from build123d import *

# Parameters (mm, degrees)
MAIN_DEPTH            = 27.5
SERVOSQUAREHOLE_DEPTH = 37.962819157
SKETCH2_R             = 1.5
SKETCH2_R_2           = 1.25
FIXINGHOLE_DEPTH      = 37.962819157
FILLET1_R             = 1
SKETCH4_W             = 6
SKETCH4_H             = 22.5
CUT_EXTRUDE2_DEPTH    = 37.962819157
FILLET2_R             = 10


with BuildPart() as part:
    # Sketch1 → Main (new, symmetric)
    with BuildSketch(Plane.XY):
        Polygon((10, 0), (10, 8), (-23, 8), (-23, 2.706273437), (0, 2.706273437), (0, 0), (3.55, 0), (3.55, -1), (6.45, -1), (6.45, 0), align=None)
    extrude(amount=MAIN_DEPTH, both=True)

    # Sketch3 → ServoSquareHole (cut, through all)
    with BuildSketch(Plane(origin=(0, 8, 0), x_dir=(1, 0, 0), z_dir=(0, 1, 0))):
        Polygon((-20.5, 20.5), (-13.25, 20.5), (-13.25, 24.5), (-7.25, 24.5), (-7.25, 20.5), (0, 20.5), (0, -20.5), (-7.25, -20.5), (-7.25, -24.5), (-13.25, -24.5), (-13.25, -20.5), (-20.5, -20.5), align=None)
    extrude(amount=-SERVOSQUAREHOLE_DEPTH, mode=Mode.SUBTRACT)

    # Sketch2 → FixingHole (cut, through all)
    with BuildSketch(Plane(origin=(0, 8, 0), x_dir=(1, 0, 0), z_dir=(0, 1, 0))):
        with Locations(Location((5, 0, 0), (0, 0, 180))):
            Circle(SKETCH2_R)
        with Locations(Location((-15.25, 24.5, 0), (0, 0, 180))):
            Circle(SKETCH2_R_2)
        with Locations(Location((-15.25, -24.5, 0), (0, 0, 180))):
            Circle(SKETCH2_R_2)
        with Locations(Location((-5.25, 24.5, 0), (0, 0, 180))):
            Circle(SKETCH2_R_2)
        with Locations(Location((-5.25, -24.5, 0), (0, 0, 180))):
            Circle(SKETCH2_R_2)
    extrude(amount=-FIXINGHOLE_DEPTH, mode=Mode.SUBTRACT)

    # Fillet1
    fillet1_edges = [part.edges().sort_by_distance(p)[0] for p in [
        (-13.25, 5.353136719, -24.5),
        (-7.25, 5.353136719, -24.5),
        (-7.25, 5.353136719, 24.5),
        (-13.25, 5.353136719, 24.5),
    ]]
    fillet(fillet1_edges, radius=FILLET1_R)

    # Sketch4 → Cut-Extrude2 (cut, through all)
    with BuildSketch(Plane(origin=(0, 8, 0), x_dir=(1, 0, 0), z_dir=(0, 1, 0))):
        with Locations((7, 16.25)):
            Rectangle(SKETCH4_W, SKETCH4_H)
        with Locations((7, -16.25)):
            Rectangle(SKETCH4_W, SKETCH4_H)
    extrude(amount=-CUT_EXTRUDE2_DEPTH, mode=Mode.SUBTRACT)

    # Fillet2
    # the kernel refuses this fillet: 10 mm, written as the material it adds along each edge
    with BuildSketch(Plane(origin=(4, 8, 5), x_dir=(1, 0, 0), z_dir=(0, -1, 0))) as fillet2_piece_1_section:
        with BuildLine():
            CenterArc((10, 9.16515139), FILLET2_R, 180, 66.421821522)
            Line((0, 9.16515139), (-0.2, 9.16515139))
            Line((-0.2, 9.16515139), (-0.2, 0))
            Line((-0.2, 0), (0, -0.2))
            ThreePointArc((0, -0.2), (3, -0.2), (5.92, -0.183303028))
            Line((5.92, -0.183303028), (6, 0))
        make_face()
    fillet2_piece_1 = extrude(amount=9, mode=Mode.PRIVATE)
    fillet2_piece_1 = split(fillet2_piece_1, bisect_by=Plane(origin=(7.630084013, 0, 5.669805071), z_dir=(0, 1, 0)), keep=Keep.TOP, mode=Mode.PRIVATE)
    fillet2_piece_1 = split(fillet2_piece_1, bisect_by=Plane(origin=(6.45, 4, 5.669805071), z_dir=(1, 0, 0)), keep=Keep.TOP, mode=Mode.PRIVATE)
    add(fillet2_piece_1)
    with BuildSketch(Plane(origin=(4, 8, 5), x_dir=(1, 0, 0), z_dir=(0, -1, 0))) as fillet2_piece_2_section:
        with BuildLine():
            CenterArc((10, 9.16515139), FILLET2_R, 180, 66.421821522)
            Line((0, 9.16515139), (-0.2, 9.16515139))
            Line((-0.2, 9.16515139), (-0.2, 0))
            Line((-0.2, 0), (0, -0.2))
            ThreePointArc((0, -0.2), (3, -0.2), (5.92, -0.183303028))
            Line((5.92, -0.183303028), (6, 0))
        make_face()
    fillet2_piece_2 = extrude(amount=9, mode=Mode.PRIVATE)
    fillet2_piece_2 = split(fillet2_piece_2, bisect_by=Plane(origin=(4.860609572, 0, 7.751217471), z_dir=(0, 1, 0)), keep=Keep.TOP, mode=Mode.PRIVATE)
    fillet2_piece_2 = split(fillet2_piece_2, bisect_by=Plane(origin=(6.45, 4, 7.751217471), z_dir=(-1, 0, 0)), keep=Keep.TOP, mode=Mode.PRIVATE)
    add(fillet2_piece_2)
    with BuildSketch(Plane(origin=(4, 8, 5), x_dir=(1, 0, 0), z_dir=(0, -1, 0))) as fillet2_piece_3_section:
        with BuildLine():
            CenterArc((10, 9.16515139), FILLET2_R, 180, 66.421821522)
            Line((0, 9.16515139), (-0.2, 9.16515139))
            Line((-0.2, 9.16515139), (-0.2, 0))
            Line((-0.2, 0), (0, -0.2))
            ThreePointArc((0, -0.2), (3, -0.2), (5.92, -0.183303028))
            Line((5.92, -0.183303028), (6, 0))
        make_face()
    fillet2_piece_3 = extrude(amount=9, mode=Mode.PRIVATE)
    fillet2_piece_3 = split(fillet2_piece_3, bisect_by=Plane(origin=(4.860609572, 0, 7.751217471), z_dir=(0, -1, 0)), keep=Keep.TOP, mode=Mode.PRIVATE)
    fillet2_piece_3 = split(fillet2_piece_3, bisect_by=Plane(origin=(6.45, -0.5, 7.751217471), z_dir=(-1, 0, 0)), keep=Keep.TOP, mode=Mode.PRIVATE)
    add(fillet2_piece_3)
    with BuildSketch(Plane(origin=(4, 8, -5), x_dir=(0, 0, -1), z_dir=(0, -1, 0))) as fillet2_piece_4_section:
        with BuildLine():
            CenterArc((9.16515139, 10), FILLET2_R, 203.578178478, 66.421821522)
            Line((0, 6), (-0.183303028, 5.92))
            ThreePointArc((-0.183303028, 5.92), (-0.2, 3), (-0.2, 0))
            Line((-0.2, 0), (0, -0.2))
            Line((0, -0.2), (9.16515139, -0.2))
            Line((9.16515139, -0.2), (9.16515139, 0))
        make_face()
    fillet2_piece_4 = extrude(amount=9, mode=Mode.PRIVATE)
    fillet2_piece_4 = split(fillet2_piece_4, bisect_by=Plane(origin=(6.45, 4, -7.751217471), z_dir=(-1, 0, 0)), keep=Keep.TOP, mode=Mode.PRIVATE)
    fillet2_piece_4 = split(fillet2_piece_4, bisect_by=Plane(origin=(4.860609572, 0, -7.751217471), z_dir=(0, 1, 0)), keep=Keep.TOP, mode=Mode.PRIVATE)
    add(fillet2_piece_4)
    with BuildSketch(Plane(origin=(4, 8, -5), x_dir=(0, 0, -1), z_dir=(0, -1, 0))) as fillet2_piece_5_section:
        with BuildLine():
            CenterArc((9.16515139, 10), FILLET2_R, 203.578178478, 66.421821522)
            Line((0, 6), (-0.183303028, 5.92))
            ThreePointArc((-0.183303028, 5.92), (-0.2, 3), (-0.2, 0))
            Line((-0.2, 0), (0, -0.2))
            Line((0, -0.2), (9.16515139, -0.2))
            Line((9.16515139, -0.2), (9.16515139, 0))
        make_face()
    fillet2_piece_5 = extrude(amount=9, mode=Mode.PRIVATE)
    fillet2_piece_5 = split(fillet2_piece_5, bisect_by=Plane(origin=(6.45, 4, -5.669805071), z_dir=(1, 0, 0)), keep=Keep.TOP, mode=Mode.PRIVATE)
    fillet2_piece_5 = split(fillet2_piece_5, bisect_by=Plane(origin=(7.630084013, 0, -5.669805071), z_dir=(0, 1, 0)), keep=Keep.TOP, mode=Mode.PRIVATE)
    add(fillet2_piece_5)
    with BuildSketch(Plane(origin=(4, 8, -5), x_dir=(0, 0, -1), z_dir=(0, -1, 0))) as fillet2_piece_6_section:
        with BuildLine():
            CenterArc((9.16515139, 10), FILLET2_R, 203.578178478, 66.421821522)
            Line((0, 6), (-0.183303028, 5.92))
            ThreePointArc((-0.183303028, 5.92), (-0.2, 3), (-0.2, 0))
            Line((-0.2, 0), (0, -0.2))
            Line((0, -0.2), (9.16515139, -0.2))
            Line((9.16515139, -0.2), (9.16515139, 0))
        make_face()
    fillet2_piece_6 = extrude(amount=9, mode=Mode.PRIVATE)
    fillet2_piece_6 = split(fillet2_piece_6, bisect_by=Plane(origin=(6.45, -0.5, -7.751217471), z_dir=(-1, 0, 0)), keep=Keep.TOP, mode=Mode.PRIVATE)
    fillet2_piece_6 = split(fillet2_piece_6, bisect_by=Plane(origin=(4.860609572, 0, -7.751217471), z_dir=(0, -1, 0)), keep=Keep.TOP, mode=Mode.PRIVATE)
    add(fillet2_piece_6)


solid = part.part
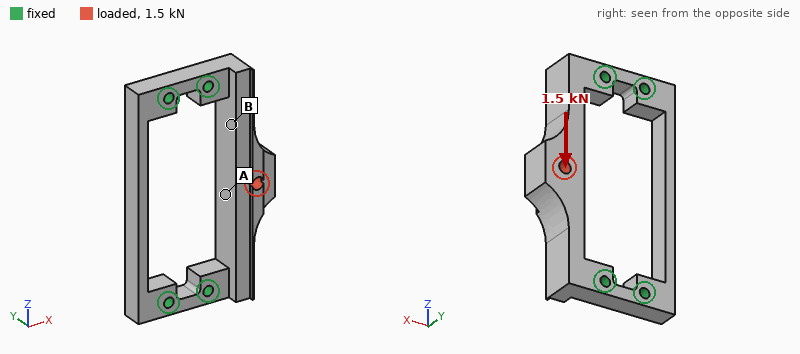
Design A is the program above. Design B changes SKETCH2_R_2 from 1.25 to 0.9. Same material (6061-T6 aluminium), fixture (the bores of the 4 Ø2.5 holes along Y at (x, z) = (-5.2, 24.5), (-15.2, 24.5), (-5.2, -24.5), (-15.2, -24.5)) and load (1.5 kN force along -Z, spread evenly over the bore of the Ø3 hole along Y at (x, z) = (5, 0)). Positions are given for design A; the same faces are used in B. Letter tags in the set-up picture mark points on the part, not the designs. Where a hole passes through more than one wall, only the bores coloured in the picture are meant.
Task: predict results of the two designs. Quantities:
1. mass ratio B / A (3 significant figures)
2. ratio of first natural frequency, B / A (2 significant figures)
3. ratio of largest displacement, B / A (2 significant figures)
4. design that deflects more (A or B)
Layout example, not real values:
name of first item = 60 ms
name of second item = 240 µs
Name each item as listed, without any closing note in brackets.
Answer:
mass ratio B / A = 1.01
ratio of first natural frequency, B / A = 0.99
ratio of largest displacement, B / A = 1.2
design that deflects more = B
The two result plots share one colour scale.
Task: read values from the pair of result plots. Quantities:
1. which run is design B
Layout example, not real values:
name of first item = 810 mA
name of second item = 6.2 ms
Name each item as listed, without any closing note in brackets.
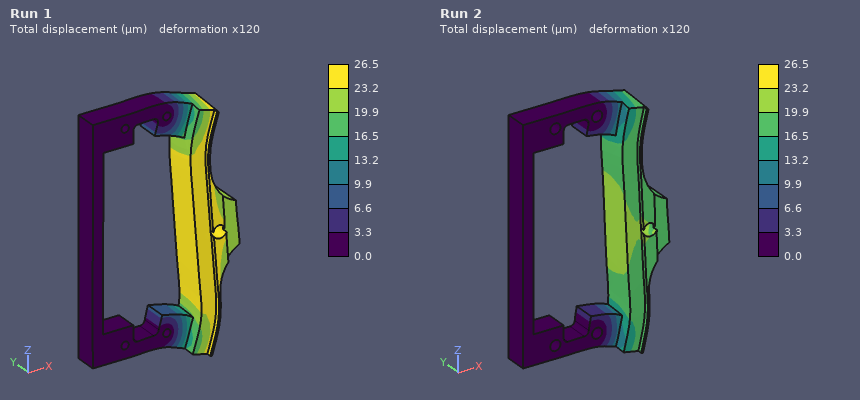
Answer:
which run is design B = Run 1
